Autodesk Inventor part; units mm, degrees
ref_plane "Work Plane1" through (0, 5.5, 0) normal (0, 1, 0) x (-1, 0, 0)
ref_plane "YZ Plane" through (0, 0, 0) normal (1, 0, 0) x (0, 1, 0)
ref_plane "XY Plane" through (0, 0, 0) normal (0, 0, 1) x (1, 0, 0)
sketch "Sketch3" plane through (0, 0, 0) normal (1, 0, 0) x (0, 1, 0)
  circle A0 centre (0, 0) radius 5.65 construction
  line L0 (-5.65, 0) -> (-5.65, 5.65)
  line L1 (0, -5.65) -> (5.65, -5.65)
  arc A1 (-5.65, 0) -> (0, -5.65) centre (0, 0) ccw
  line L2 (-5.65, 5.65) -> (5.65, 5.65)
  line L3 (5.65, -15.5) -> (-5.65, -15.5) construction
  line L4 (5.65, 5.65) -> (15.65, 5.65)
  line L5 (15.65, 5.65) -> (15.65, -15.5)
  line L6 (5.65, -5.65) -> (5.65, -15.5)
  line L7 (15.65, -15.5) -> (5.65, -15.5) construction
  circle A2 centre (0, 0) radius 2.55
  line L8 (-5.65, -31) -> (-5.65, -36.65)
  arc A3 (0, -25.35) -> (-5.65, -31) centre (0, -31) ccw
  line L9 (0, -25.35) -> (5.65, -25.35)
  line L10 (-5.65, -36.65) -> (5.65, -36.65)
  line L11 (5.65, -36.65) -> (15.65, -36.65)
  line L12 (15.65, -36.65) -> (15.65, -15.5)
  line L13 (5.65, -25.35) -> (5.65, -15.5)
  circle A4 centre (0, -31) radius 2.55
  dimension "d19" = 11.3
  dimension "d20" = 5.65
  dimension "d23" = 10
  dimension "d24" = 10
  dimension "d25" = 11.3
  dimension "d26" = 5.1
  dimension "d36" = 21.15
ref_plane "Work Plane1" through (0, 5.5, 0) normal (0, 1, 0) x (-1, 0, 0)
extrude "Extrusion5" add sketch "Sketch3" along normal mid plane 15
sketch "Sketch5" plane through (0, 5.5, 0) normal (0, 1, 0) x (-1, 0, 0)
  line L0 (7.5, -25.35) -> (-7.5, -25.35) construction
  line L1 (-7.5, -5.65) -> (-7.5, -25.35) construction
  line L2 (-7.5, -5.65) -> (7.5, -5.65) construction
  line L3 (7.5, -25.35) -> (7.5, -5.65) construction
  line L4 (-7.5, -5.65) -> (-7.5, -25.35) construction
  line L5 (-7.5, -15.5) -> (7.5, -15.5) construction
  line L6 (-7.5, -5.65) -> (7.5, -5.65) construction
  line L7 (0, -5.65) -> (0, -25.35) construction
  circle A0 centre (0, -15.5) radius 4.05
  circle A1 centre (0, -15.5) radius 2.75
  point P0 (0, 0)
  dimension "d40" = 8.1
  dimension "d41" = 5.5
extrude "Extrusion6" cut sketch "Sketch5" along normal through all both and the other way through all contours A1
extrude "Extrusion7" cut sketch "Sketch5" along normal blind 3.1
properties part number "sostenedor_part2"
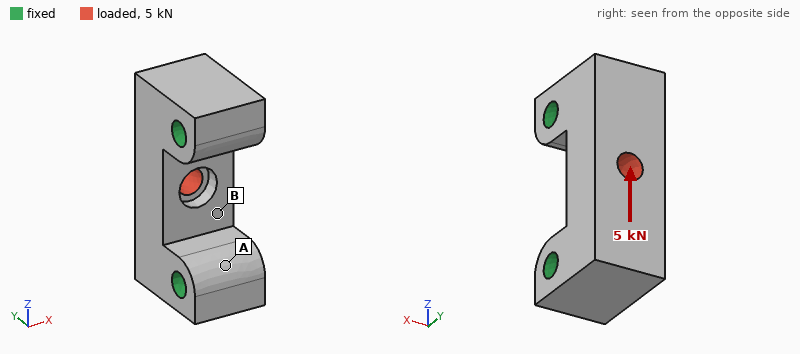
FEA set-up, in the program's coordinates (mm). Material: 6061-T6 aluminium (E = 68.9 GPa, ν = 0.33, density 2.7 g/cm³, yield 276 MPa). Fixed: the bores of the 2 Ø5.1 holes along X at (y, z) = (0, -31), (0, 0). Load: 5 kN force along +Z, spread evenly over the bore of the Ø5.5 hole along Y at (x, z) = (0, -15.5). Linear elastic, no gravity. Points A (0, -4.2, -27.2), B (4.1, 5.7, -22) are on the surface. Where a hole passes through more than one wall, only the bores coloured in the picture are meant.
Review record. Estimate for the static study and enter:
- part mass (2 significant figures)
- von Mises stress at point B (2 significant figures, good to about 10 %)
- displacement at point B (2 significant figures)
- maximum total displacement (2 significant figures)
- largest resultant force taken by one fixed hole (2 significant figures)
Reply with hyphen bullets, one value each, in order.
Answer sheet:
- 24 g
- 33 MPa
- 8.3 µm
- 13 µm
- 2.7 kN
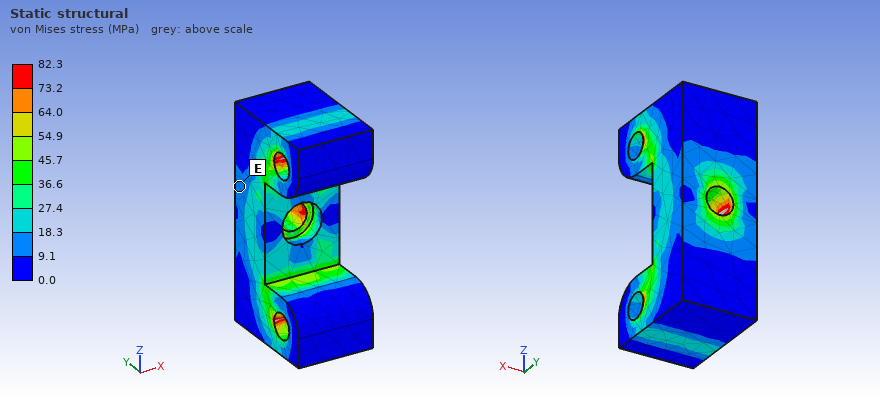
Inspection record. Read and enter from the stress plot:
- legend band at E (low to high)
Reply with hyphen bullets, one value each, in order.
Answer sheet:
- 9.1 to 18.3 MPa
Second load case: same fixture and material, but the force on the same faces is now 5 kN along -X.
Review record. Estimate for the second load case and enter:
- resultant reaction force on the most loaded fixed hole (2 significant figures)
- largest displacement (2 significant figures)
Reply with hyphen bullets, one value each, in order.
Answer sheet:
- 2.5 kN
- 33 µm
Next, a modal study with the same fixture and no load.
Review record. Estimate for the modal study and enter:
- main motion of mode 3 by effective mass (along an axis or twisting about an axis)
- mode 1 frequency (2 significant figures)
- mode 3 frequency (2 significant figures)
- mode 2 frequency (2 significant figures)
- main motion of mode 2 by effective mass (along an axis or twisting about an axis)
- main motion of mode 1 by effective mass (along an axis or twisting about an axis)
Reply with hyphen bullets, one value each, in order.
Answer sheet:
- twisting about Y
- 26 kHz
- 36 kHz
- 29 kHz
- along Z
- along X
